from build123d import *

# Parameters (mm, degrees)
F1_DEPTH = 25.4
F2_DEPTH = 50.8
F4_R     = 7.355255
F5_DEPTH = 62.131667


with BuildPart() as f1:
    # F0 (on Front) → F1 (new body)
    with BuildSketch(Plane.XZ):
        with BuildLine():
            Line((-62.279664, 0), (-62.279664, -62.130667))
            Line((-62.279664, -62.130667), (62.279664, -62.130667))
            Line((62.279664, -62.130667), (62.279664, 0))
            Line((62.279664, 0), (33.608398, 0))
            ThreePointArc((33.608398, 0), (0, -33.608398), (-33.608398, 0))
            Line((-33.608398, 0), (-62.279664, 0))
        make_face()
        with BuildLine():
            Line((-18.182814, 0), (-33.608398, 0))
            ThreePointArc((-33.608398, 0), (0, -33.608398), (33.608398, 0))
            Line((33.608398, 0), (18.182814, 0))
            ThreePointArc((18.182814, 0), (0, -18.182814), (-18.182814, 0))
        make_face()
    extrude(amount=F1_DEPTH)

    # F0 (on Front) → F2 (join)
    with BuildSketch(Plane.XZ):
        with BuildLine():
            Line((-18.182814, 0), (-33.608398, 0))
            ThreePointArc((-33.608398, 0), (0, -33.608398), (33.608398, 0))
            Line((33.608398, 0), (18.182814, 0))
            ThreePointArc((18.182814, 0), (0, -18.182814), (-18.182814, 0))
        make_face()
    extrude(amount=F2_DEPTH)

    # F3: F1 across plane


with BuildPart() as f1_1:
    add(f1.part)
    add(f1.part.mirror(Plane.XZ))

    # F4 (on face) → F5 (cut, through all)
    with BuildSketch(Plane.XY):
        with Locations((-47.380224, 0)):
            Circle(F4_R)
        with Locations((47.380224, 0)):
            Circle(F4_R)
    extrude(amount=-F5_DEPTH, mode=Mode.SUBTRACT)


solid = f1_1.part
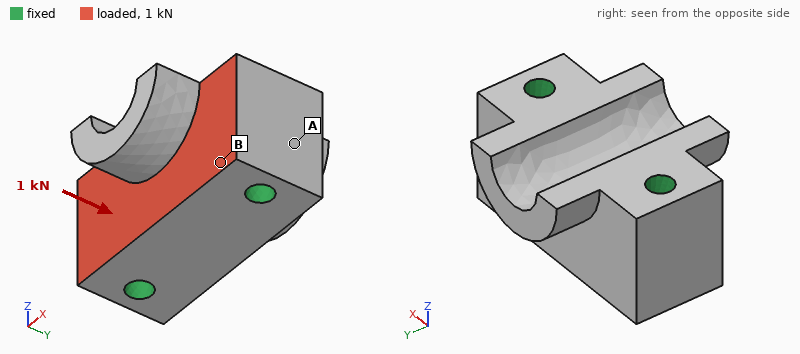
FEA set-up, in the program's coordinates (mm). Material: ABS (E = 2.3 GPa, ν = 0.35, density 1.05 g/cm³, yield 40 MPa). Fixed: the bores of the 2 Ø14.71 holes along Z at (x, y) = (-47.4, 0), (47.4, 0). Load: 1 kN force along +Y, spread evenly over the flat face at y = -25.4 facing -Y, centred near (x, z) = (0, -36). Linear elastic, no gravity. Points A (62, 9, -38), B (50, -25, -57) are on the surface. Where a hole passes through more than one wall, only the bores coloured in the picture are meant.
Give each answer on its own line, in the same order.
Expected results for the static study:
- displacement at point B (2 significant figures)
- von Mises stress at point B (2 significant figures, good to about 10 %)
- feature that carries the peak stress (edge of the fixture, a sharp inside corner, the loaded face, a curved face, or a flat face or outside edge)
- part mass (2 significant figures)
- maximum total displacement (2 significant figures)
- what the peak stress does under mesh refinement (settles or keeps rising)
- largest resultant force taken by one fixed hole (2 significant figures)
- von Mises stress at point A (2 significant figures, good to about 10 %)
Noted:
2.1 µm
0.23 MPa
edge of the fixture
430 g
8.0 µm
keeps rising
500 N
0.077 MPa
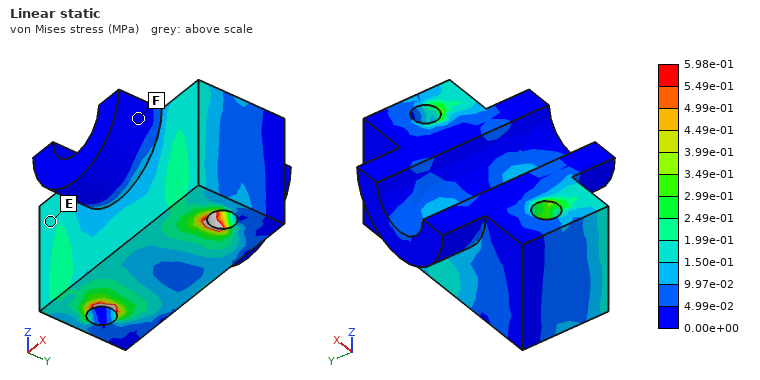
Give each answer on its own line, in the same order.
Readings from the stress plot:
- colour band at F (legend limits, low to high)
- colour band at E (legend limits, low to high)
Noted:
0.00e+00 to 4.99e-02 MPa
1.50e-01 to 1.99e-01 MPa
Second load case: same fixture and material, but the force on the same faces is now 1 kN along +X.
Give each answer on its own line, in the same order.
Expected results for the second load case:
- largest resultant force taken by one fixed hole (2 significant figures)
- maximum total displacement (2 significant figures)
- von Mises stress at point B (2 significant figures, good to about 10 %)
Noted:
540 N
9.2 µm
0.36 MPa
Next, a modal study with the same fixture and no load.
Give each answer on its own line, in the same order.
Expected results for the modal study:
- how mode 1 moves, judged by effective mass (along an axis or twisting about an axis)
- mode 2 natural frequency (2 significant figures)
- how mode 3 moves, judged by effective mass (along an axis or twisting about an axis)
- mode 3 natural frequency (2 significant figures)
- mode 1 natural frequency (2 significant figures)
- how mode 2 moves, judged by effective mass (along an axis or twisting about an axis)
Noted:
twisting about X
3200 Hz
along Y
3400 Hz
2900 Hz
along Z
